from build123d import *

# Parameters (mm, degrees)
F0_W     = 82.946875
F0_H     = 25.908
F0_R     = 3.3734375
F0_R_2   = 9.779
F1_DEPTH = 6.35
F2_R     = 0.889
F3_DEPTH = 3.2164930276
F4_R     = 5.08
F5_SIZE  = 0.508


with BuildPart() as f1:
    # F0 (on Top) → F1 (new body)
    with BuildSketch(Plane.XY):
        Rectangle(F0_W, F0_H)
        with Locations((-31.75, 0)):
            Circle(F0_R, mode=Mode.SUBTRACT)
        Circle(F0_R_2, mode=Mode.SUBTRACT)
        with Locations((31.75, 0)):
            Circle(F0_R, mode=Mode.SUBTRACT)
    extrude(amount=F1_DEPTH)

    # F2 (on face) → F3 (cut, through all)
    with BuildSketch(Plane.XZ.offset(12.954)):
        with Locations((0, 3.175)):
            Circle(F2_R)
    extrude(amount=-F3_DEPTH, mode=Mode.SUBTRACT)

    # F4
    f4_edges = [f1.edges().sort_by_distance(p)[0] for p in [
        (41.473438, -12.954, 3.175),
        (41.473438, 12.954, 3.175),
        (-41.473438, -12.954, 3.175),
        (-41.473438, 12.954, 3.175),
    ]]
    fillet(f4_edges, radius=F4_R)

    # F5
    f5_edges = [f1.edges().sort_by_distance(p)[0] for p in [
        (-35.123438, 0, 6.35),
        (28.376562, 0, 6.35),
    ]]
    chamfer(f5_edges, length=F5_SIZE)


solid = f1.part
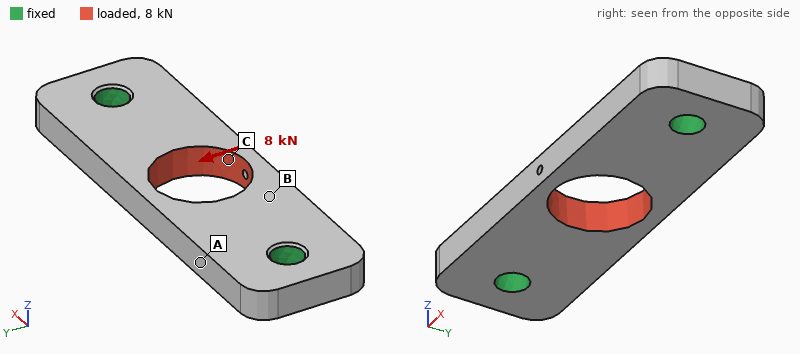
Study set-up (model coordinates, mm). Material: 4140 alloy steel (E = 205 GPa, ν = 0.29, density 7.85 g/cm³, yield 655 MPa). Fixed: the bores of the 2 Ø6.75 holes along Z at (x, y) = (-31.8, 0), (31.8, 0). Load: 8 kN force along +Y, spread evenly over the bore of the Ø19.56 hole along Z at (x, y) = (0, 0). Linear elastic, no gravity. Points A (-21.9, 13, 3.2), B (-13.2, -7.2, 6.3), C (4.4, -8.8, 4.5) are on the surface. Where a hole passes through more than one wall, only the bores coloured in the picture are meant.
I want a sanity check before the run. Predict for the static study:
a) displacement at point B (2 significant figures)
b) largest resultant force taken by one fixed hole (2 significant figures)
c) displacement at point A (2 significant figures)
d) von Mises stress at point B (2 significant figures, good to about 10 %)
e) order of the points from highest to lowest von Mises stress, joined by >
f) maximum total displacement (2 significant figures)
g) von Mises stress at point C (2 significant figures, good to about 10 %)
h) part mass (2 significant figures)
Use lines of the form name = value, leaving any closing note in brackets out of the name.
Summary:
displacement at point B = 16 µm
largest resultant force taken by one fixed hole = 4.0 kN
displacement at point A = 11 µm
von Mises stress at point B = 52 MPa
order of the points from highest to lowest von Mises stress, joined by > = C > B > A
maximum total displacement = 25 µm
von Mises stress at point C = 95 MPa
part mass = 87 g
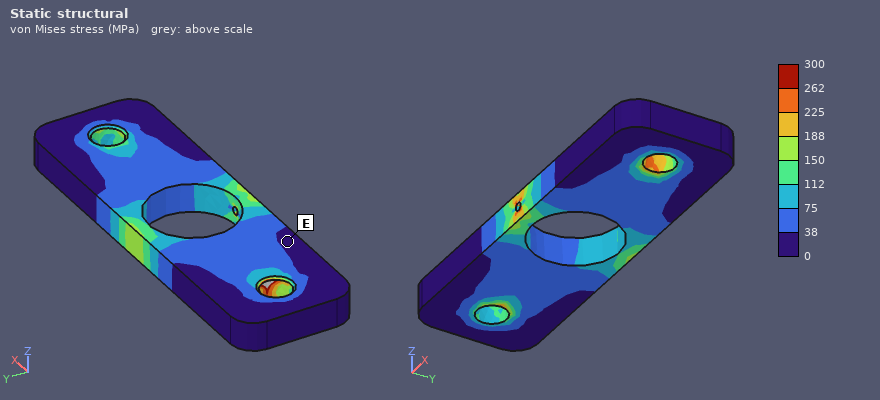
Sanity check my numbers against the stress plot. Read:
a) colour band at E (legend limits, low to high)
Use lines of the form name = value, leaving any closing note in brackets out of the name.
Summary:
colour band at E = 0 to 38 MPa
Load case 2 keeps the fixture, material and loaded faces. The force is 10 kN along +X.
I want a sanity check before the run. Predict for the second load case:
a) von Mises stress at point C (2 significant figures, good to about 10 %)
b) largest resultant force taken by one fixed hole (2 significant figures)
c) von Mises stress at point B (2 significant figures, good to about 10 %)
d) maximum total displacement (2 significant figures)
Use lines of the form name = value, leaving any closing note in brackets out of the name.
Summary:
von Mises stress at point C = 55 MPa
largest resultant force taken by one fixed hole = 5.0 kN
von Mises stress at point B = 35 MPa
maximum total displacement = 5.8 µm
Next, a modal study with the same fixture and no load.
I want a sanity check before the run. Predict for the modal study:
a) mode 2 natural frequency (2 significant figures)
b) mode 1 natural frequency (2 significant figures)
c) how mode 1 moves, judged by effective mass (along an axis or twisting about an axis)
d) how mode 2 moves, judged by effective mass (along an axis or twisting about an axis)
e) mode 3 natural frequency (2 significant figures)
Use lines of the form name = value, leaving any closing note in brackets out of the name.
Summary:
mode 2 natural frequency = 12 kHz
mode 1 natural frequency = 8800 Hz
how mode 1 moves, judged by effective mass = along Z
how mode 2 moves, judged by effective mass = twisting about X
mode 3 natural frequency = 18 kHz
